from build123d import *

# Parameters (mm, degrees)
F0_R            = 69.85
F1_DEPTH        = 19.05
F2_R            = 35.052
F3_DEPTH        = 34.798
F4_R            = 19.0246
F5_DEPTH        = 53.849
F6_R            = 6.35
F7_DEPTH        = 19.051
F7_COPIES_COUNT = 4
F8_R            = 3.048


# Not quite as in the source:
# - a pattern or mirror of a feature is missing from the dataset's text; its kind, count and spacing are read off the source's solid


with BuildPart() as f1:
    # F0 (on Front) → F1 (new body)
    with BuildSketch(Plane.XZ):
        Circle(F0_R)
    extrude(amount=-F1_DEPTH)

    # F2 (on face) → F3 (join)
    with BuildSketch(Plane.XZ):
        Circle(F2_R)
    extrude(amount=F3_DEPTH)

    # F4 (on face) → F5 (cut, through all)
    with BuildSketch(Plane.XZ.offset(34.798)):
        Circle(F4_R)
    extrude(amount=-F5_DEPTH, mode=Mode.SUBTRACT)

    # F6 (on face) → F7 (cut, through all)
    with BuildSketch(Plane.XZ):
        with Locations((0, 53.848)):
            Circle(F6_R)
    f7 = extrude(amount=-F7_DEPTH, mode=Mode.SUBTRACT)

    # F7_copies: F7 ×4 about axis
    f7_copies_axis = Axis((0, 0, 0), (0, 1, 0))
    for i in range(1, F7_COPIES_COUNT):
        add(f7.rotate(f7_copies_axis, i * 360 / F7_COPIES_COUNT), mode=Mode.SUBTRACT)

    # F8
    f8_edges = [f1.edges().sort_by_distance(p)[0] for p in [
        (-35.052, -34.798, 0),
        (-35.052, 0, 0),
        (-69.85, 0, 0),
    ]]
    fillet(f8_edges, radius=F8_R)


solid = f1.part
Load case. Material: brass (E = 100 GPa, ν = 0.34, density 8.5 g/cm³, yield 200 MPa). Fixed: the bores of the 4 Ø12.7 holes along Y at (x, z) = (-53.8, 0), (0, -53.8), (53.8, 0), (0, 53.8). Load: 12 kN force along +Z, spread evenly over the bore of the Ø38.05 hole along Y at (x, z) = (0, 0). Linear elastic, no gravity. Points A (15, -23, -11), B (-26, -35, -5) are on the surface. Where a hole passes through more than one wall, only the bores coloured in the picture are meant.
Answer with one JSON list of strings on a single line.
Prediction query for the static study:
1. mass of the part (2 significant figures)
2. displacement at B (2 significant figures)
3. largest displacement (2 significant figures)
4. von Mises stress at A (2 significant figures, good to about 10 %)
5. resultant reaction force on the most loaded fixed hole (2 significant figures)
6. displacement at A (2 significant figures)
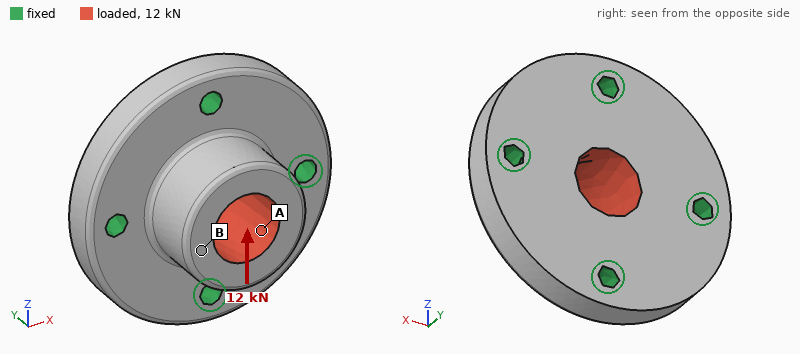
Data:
["3.0 kg", "5.7 µm", "6.9 µm", "5.2 MPa", "4.3 kN", "5.2 µm"]
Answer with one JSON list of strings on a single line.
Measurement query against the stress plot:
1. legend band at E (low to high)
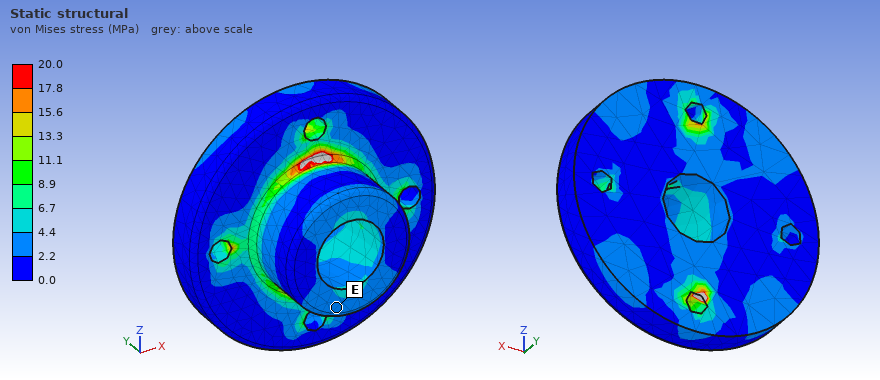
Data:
["2.2 to 4.4 MPa"]
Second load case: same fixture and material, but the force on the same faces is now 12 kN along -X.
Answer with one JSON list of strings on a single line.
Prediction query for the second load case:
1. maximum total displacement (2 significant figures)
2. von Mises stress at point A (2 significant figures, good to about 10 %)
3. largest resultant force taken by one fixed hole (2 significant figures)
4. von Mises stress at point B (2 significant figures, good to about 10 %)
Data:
["6.9 µm", "4.4 MPa", "4.3 kN", "4.0 MPa"]
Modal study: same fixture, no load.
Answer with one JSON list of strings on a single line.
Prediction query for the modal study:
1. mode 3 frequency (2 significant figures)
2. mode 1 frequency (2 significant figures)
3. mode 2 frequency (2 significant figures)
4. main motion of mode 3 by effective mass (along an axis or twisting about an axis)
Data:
["6600 Hz", "6300 Hz", "6300 Hz", "along Y"]
